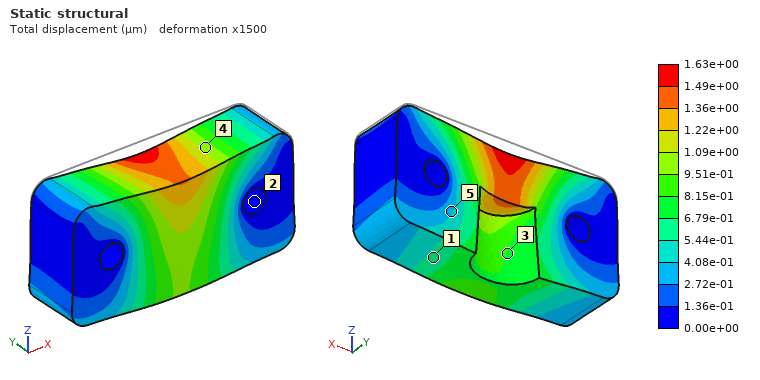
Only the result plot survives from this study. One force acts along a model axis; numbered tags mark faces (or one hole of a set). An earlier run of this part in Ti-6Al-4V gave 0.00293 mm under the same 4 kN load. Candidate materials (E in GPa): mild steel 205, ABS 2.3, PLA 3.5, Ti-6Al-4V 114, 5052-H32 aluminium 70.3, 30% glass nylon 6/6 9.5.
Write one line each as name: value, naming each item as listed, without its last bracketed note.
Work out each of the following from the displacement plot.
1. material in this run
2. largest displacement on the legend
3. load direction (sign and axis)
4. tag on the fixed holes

material in this run: mild steel
largest displacement on the legend: 1.63e+00 µm
load direction: -Z
tag on the fixed holes: 2
